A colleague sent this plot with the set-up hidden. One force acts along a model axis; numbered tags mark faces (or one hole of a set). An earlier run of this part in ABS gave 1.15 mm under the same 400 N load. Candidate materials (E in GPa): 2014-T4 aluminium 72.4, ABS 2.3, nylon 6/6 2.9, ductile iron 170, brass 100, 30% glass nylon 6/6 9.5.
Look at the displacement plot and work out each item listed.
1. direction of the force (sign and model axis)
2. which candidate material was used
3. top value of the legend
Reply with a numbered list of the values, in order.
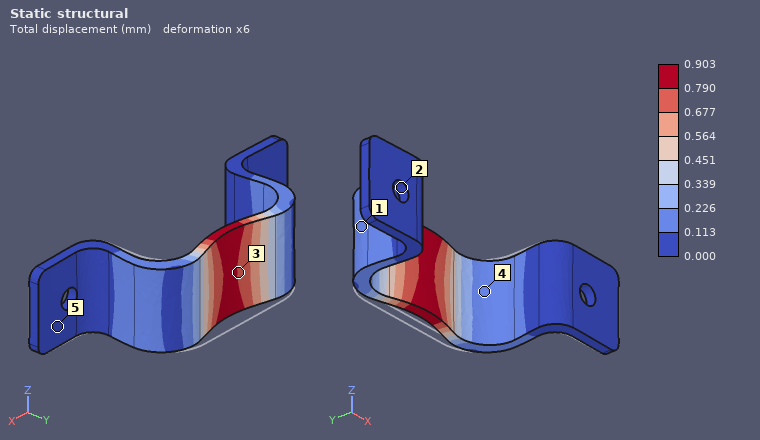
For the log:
1. -Y
2. nylon 6/6
3. 0.903 mm
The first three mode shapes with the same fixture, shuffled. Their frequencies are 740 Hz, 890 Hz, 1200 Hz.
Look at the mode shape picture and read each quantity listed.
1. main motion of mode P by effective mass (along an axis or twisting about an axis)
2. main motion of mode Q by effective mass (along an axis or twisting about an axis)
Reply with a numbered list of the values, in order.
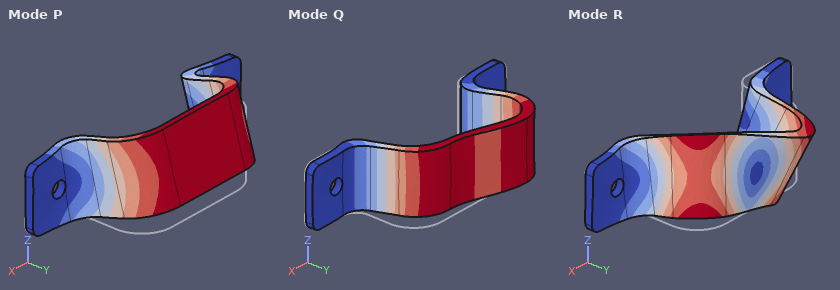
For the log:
1. along Z
2. along X
